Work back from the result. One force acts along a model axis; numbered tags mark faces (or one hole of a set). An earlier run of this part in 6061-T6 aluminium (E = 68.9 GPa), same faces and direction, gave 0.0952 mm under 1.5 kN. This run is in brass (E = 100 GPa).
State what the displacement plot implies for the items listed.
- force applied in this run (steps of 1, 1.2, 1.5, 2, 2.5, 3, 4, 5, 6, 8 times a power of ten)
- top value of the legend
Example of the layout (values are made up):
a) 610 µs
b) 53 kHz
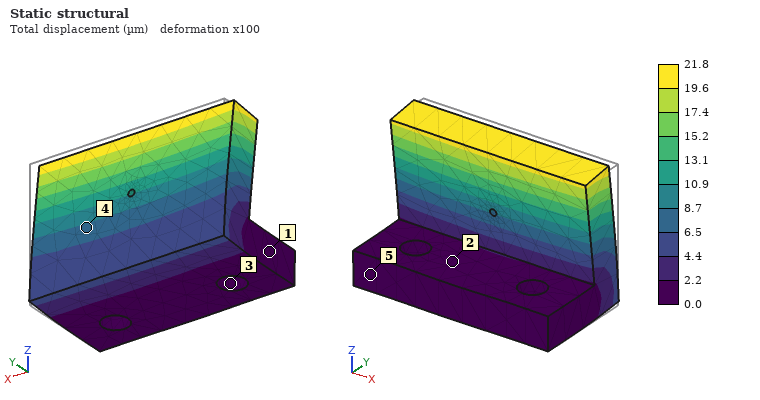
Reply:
a) 500 N
b) 21.8 µm
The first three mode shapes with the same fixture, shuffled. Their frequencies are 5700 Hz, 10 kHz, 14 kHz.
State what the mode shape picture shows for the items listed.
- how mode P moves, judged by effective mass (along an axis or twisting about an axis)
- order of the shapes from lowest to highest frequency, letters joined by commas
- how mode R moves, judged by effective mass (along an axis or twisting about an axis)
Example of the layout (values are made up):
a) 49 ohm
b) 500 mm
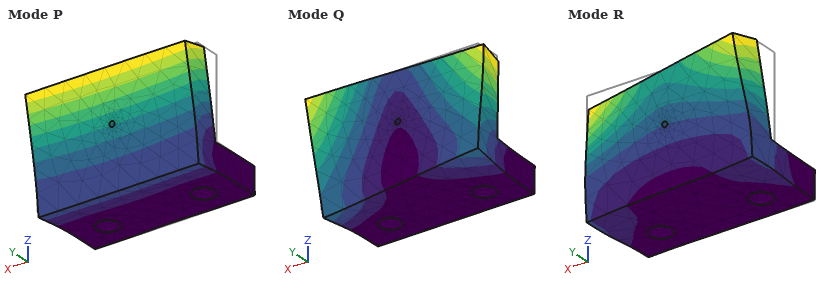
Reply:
a) along Y
b) P, Q, R
c) along X
